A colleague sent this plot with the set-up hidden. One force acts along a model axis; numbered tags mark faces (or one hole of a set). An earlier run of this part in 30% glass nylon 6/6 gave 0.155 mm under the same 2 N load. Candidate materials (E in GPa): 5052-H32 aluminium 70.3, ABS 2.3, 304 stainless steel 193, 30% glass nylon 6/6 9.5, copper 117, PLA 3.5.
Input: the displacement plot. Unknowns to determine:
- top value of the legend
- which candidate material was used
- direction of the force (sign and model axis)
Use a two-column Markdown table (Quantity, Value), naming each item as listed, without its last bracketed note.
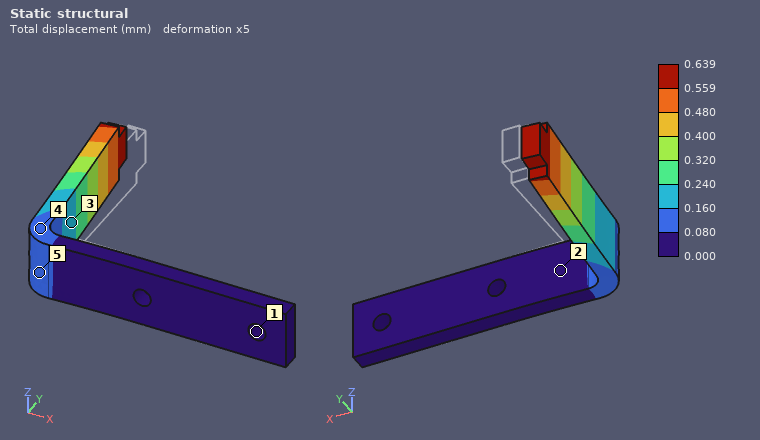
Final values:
| Quantity | Value |
|---|---|
| top value of the legend | 0.639 mm |
| which candidate material was used | ABS |
| direction of the force | -X |
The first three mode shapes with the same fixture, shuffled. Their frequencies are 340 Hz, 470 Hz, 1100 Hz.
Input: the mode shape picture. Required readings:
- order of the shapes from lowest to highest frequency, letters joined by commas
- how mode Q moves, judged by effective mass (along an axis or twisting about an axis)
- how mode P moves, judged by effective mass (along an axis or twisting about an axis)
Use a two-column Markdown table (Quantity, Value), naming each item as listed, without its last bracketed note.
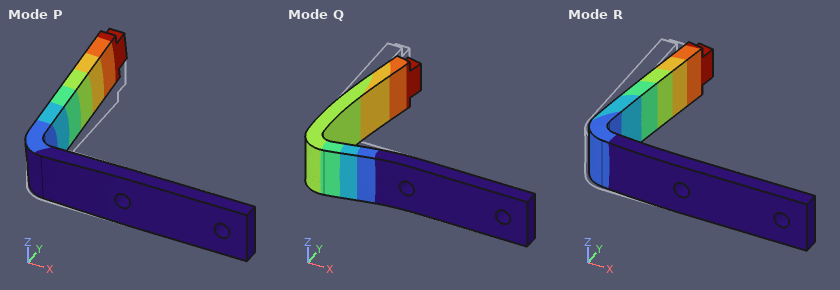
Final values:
| Quantity | Value |
|---|---|
| order of the shapes from lowest to highest frequency, letters joined by commas | R, P, Q |
| how mode Q moves, judged by effective mass | along Y |
| how mode P moves, judged by effective mass | along Z |
